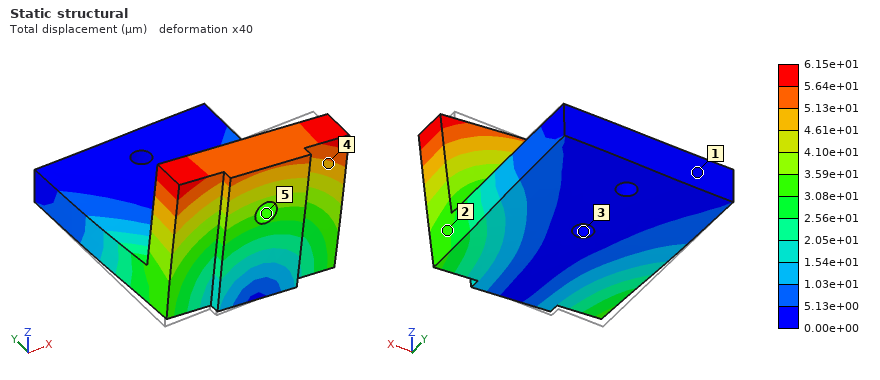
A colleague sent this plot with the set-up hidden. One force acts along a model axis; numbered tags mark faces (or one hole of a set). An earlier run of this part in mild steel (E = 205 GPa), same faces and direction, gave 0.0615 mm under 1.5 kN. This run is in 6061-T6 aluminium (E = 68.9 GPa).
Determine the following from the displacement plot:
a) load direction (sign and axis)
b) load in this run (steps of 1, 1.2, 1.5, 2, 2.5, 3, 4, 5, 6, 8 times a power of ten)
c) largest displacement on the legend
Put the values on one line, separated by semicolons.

+X; 500 N; 6.15e+01 µm
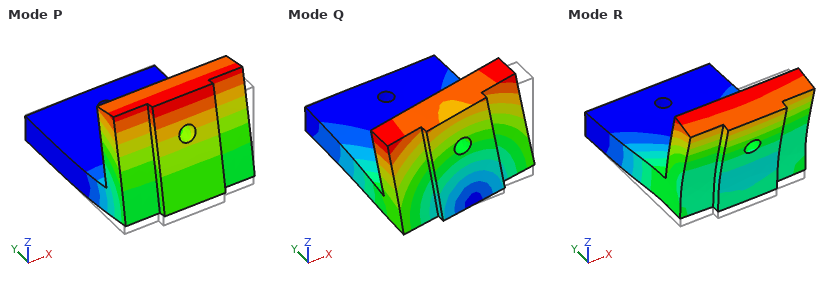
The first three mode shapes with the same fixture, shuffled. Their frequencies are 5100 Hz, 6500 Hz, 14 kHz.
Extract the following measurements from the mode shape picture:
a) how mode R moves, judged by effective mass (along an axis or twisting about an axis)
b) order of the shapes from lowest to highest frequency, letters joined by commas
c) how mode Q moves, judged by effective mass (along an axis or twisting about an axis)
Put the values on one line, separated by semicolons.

along Z; P, Q, R; along X
